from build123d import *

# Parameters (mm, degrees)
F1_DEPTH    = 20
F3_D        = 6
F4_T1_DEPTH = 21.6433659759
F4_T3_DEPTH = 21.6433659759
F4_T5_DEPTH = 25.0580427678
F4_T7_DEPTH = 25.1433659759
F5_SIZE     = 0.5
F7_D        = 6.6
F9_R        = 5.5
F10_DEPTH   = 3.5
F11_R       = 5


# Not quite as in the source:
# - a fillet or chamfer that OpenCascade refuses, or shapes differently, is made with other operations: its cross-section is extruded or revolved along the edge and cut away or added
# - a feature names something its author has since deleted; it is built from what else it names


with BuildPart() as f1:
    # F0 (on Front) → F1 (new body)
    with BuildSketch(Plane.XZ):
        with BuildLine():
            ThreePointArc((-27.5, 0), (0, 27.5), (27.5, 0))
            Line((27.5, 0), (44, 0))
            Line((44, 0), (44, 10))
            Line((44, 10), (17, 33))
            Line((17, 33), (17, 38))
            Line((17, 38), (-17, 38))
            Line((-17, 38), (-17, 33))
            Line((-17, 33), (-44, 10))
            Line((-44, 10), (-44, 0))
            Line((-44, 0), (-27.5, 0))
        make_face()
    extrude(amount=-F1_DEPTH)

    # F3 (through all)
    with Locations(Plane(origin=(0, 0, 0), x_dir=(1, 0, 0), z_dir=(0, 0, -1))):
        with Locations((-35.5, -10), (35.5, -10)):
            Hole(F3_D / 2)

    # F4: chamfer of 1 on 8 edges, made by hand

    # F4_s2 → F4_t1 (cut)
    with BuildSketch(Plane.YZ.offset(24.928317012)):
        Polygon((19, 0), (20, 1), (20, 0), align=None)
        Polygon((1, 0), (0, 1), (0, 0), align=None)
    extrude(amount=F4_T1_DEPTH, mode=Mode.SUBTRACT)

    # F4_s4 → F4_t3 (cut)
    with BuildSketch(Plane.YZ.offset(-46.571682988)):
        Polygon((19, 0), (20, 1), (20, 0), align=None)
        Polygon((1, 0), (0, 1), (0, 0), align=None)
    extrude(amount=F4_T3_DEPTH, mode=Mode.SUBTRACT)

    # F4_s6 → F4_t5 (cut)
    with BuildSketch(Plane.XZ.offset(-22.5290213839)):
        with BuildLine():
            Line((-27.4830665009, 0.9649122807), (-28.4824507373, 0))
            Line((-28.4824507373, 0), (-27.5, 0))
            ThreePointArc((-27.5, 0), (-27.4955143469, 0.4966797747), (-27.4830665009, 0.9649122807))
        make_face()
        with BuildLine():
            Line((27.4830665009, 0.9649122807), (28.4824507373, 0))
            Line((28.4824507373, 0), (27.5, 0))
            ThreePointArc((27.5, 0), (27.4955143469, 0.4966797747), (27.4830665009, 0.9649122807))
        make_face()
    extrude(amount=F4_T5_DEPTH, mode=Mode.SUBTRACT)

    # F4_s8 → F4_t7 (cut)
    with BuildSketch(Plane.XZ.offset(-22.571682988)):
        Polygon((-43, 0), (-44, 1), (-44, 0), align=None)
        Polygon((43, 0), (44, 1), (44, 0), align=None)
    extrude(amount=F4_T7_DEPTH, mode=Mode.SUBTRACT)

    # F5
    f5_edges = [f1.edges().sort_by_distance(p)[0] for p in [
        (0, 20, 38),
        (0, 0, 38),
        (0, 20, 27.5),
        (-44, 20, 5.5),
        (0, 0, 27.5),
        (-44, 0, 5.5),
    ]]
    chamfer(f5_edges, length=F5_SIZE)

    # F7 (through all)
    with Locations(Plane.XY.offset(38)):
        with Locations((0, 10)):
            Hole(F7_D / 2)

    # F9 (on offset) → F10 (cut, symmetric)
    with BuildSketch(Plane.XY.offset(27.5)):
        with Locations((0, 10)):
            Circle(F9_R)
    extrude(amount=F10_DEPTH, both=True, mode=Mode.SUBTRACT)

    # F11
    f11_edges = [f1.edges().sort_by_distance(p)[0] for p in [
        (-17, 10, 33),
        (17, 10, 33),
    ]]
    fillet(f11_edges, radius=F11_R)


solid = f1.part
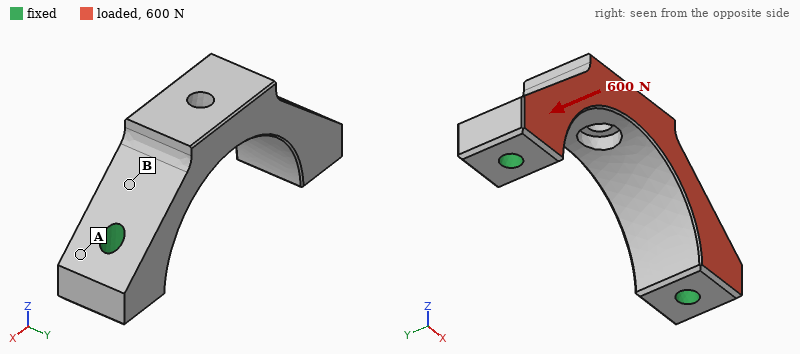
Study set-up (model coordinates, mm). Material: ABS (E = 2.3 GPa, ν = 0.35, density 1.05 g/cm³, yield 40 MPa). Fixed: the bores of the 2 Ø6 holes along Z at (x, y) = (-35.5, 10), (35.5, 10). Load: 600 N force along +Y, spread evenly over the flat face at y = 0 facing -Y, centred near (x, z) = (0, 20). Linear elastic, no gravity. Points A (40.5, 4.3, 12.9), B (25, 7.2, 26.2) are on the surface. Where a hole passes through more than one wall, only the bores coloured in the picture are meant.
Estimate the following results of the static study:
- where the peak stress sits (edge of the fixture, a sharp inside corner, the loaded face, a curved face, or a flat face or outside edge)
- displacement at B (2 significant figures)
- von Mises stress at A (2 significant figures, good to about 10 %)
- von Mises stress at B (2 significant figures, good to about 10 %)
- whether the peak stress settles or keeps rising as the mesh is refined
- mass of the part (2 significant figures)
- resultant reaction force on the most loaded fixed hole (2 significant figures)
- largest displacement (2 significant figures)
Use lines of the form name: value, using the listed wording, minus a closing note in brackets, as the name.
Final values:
where the peak stress sits: edge of the fixture
displacement at B: 0.059 mm
von Mises stress at A: 1.7 MPa
von Mises stress at B: 3.5 MPa
whether the peak stress settles or keeps rising as the mesh is refined: keeps rising
mass of the part: 25 g
resultant reaction force on the most loaded fixed hole: 300 N
largest displacement: 0.16 mm
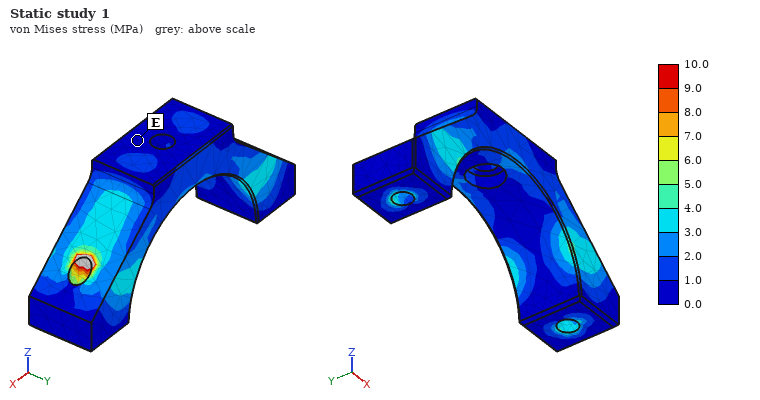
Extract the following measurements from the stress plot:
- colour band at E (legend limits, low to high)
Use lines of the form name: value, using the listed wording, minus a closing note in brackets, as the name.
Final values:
colour band at E: 0.0 to 1.0 MPa
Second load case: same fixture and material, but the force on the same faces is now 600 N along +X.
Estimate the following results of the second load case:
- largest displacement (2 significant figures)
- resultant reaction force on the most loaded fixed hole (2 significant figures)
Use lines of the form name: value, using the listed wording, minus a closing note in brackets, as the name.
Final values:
largest displacement: 47 µm
resultant reaction force on the most loaded fixed hole: 310 N
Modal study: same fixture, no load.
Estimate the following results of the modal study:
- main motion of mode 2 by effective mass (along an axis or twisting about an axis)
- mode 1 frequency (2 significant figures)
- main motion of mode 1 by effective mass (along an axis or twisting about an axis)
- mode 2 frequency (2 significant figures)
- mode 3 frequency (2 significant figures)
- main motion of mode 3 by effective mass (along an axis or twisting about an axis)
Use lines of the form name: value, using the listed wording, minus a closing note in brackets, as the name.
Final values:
main motion of mode 2 by effective mass: along X
mode 1 frequency: 2400 Hz
main motion of mode 1 by effective mass: along Y
mode 2 frequency: 4800 Hz
mode 3 frequency: 5400 Hz
main motion of mode 3 by effective mass: along Z
